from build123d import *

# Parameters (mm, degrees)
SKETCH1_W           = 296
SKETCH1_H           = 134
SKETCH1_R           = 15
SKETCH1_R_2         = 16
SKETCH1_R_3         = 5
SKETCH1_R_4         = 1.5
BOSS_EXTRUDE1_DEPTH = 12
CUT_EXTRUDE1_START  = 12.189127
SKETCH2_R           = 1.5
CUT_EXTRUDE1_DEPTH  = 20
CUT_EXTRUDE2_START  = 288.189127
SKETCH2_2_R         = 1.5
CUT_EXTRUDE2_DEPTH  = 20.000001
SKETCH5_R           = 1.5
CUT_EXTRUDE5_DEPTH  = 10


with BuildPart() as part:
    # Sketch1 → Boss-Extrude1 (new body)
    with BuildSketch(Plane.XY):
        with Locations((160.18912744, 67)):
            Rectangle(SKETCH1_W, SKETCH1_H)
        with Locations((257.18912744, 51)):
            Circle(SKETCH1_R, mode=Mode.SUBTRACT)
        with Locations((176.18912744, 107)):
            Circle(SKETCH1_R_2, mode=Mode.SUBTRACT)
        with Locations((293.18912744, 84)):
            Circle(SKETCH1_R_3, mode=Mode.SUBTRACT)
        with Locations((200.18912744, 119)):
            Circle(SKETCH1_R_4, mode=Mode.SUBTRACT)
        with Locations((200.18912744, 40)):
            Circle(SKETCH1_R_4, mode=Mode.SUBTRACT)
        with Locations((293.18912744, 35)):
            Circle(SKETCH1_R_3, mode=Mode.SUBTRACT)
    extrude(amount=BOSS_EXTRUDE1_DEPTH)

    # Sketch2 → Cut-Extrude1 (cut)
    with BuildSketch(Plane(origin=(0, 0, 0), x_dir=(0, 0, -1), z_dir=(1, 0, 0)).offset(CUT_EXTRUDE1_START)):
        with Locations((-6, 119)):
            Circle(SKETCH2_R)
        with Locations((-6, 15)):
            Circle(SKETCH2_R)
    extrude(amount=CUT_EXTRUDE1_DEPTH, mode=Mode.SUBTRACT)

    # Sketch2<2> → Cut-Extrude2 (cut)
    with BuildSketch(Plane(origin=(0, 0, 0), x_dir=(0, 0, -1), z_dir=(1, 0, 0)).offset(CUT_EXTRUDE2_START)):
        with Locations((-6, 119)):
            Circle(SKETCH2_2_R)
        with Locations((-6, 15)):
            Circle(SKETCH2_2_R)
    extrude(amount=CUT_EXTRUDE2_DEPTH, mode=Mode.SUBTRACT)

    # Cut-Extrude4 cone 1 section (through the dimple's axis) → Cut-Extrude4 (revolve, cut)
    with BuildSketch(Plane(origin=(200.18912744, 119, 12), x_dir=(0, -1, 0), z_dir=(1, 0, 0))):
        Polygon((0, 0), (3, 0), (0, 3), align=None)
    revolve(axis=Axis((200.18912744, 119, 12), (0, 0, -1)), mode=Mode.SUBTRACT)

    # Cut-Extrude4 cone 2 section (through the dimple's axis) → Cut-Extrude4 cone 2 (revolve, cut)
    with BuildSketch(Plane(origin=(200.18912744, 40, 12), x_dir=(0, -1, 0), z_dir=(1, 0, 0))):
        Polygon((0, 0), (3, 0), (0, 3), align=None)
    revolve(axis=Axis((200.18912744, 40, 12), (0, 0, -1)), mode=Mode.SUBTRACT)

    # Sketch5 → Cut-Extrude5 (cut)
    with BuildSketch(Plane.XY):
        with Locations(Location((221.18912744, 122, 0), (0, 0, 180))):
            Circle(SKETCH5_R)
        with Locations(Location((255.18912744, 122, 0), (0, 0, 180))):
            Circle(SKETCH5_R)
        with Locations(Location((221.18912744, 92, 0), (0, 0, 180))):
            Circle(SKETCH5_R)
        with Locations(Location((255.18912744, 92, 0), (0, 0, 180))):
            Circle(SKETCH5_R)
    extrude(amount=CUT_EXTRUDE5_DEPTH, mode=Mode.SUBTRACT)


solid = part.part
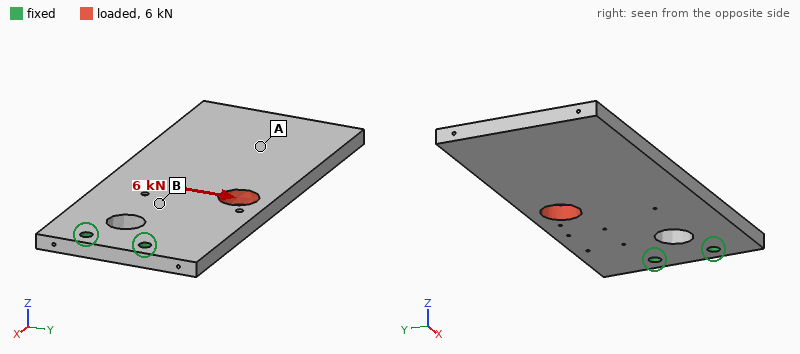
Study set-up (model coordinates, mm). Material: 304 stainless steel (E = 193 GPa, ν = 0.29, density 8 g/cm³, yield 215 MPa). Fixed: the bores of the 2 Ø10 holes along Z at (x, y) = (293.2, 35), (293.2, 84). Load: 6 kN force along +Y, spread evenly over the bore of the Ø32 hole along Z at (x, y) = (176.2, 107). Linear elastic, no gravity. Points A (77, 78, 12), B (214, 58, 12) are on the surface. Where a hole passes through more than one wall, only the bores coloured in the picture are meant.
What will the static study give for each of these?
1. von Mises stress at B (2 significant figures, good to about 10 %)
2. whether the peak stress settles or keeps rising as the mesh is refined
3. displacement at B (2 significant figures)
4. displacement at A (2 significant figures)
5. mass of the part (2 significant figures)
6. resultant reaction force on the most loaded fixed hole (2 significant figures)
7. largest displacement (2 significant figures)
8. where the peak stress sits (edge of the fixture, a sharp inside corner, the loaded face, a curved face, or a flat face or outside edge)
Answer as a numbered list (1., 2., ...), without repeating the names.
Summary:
1. 13 MPa
2. keeps rising
3. 28 µm
4. 71 µm
5. 3.6 kg
6. 12 kN
7. 93 µm
8. edge of the fixture
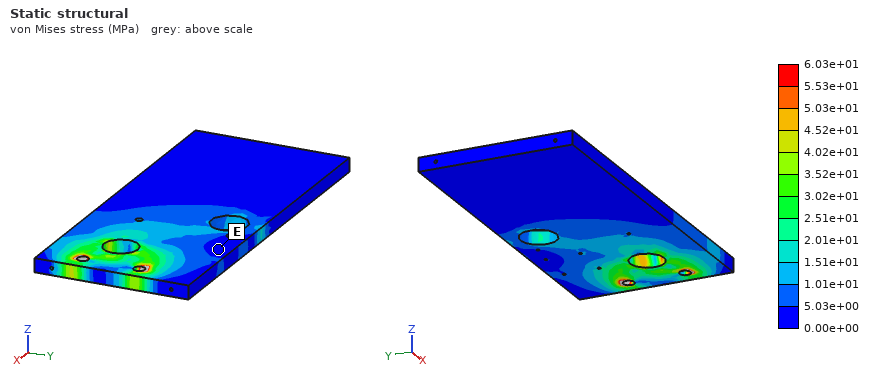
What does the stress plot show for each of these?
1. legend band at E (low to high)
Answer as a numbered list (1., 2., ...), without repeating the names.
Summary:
1. 0.00e+00 to 5.03e+00 MPa
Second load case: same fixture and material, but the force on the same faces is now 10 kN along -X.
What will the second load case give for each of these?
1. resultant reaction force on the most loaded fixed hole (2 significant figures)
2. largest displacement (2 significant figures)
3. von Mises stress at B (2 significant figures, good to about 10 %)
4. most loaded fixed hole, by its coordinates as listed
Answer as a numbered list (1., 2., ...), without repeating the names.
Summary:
1. 13 kN
2. 66 µm
3. 6.5 MPa
4. (293.2, 84)
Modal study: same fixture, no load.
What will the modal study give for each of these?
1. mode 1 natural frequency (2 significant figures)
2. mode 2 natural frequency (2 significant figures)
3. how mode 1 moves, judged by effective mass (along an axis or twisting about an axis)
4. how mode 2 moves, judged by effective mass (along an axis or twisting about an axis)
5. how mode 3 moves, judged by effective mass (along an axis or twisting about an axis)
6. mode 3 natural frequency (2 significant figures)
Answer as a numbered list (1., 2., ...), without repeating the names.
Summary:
1. 110 Hz
2. 480 Hz
3. along Z
4. twisting about X
5. along Z
6. 710 Hz
